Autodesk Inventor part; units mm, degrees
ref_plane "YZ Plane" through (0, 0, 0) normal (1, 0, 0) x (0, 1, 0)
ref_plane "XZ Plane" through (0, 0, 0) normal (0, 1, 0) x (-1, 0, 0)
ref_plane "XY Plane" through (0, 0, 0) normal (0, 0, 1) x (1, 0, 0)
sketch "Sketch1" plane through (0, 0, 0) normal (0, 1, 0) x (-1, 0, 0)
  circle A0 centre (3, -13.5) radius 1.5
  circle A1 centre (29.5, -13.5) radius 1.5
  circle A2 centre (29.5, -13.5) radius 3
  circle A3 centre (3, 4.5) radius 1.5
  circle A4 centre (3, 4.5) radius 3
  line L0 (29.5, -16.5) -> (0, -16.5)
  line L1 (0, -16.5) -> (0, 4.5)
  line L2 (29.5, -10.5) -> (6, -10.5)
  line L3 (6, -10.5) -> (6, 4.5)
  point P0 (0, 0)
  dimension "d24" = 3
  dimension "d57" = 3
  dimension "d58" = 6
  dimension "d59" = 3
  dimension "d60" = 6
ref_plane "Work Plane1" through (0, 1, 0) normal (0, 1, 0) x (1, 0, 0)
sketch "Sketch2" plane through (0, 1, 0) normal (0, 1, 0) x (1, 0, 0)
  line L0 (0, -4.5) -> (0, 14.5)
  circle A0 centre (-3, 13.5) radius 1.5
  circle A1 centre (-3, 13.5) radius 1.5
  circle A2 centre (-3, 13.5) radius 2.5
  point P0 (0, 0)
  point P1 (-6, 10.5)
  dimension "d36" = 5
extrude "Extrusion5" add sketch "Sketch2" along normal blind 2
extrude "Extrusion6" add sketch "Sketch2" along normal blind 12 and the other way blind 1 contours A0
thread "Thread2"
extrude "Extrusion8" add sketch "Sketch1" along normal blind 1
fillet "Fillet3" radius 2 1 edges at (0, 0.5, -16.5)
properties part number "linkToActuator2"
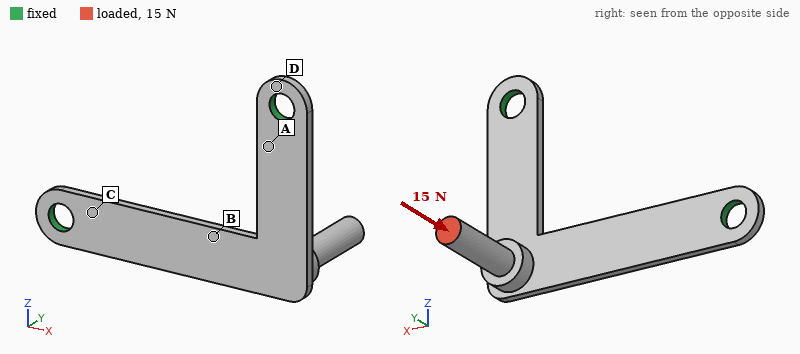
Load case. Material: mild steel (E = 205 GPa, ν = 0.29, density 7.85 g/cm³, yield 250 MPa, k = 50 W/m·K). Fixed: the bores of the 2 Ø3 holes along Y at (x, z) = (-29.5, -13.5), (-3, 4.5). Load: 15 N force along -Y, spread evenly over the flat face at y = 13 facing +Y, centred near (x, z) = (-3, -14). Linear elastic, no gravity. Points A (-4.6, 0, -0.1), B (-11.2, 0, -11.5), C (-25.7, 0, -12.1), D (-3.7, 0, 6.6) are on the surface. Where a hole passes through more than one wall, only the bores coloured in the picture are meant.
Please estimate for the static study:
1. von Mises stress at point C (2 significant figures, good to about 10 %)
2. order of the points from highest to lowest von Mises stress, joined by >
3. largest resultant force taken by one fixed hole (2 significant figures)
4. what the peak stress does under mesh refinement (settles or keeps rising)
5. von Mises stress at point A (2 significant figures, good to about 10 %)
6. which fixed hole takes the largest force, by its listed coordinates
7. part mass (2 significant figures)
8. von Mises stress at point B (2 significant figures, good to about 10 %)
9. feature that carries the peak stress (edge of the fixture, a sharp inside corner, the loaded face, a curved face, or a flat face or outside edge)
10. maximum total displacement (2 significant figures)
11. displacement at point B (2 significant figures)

68 MPa
A > C > B > D
11 N
keeps rising
99 MPa
(-3, 4.5)
3.1 g
42 MPa
edge of the fixture
0.15 mm
0.050 mm
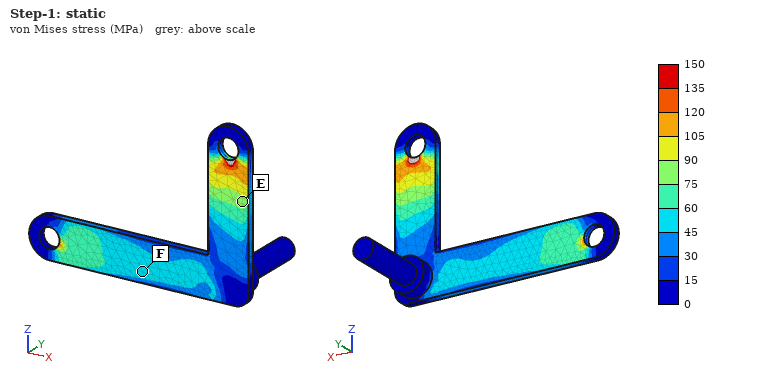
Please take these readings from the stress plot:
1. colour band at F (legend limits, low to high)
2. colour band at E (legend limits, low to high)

45 to 60 MPa
75 to 90 MPa
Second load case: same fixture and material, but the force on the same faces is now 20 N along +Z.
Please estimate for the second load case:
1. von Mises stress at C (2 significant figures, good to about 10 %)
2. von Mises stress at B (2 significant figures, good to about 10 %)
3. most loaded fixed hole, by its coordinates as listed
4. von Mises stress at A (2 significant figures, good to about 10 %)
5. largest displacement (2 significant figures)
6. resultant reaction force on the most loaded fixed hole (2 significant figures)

110 MPa
83 MPa
(-3, 4.5)
91 MPa
0.26 mm
21 N
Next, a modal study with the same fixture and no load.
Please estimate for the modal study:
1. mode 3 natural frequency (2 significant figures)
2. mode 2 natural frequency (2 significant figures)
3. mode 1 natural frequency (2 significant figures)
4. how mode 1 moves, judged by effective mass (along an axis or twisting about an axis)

5200 Hz
3900 Hz
1500 Hz
along Y
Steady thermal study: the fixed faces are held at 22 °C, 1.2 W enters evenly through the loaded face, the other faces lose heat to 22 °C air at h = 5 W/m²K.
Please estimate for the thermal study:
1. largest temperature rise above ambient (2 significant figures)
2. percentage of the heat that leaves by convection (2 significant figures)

74 K
7.3 %
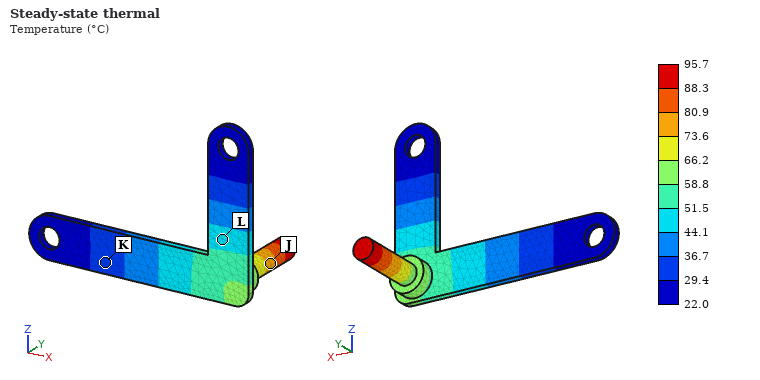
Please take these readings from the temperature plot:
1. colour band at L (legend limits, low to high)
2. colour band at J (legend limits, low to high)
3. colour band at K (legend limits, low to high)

44.1 to 51.5 °C
73.6 to 80.9 °C
29.4 to 36.7 °C
